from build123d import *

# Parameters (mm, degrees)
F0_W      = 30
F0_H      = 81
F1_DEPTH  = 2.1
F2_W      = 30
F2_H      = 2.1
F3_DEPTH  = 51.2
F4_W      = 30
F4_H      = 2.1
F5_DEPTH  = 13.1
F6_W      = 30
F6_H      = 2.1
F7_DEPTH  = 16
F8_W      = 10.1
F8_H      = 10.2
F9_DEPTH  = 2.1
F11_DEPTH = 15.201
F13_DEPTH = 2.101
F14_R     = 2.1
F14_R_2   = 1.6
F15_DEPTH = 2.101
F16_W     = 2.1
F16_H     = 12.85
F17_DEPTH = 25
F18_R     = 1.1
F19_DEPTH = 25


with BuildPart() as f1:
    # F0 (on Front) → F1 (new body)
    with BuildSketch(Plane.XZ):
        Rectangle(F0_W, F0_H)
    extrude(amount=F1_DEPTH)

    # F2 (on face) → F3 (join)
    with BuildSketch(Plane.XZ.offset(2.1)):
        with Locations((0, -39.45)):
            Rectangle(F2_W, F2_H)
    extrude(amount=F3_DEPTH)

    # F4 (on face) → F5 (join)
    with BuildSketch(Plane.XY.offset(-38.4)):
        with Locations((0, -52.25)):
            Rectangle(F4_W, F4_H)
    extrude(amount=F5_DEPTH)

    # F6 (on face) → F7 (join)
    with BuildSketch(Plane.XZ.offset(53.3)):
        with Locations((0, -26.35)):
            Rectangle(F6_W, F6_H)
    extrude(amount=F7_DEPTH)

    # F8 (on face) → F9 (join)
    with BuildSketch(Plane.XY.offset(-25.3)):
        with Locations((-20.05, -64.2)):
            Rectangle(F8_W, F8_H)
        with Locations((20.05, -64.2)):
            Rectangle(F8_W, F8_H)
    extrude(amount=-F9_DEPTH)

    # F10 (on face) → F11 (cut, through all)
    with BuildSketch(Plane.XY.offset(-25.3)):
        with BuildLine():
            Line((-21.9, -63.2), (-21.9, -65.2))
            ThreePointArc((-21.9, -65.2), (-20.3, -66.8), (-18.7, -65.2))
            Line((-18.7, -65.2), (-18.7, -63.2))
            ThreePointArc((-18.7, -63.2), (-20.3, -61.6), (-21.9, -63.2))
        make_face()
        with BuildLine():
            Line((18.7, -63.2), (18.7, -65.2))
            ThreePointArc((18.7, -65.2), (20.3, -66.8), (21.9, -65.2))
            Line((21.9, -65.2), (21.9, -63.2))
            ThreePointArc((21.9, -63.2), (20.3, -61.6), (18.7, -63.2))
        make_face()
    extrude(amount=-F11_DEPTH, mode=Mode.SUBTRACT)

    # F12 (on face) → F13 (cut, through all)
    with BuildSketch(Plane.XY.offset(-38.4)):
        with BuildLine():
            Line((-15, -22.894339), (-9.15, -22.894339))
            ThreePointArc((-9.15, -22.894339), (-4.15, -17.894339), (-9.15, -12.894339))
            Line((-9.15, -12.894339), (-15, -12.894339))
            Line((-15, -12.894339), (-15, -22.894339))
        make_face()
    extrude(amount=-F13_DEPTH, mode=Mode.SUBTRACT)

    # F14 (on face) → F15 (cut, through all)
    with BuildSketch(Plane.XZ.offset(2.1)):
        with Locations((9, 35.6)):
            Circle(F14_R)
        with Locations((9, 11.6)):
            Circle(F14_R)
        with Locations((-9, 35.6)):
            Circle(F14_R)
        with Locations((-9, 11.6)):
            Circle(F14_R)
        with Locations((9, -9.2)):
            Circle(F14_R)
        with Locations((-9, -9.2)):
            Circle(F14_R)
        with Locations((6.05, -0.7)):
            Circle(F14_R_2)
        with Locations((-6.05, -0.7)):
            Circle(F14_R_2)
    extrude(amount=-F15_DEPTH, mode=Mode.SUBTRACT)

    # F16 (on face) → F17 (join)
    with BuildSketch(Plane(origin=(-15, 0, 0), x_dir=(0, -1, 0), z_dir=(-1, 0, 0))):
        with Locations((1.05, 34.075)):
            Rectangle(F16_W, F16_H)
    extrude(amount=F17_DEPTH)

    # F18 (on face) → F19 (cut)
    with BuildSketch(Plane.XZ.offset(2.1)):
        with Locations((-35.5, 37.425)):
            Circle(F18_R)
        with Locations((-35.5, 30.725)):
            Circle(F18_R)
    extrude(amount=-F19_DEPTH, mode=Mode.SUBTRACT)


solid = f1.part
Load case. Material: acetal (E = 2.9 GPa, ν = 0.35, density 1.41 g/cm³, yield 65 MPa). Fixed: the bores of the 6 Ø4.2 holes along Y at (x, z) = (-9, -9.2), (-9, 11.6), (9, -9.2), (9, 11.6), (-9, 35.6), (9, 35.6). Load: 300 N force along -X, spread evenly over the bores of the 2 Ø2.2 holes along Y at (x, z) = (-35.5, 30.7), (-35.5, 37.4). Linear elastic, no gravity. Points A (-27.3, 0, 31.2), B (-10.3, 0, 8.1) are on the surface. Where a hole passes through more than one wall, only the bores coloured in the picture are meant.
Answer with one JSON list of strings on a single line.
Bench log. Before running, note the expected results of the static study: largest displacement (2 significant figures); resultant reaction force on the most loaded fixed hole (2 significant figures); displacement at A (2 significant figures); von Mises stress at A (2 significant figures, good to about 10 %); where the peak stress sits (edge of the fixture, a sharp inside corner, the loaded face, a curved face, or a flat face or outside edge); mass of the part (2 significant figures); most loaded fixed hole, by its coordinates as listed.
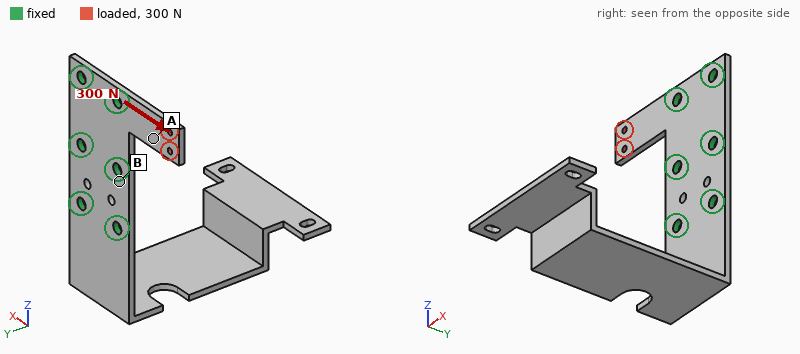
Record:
["0.11 mm", "250 N", "0.070 mm", "11 MPa", "the loaded face", "15 g", "(-9, 35.6)"]
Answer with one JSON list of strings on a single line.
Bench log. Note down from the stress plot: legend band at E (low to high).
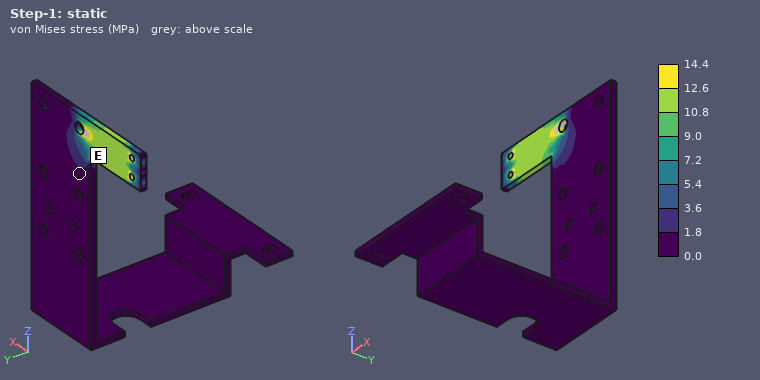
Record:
["0.0 to 1.8 MPa"]
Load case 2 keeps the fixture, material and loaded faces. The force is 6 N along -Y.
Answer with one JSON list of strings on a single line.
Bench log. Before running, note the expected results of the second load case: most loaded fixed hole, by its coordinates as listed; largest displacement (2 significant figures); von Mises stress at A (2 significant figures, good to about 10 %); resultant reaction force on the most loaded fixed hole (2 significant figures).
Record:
["(-9, 35.6)", "1.3 mm", "5.2 MPa", "7.5 N"]
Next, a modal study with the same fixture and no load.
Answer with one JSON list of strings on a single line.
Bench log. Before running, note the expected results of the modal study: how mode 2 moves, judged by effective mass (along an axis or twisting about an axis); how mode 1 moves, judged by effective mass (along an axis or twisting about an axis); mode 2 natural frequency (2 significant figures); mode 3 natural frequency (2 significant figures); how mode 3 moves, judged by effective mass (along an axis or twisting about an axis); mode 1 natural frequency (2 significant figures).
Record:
["along X", "along Z", "88 Hz", "180 Hz", "along Y", "49 Hz"]
